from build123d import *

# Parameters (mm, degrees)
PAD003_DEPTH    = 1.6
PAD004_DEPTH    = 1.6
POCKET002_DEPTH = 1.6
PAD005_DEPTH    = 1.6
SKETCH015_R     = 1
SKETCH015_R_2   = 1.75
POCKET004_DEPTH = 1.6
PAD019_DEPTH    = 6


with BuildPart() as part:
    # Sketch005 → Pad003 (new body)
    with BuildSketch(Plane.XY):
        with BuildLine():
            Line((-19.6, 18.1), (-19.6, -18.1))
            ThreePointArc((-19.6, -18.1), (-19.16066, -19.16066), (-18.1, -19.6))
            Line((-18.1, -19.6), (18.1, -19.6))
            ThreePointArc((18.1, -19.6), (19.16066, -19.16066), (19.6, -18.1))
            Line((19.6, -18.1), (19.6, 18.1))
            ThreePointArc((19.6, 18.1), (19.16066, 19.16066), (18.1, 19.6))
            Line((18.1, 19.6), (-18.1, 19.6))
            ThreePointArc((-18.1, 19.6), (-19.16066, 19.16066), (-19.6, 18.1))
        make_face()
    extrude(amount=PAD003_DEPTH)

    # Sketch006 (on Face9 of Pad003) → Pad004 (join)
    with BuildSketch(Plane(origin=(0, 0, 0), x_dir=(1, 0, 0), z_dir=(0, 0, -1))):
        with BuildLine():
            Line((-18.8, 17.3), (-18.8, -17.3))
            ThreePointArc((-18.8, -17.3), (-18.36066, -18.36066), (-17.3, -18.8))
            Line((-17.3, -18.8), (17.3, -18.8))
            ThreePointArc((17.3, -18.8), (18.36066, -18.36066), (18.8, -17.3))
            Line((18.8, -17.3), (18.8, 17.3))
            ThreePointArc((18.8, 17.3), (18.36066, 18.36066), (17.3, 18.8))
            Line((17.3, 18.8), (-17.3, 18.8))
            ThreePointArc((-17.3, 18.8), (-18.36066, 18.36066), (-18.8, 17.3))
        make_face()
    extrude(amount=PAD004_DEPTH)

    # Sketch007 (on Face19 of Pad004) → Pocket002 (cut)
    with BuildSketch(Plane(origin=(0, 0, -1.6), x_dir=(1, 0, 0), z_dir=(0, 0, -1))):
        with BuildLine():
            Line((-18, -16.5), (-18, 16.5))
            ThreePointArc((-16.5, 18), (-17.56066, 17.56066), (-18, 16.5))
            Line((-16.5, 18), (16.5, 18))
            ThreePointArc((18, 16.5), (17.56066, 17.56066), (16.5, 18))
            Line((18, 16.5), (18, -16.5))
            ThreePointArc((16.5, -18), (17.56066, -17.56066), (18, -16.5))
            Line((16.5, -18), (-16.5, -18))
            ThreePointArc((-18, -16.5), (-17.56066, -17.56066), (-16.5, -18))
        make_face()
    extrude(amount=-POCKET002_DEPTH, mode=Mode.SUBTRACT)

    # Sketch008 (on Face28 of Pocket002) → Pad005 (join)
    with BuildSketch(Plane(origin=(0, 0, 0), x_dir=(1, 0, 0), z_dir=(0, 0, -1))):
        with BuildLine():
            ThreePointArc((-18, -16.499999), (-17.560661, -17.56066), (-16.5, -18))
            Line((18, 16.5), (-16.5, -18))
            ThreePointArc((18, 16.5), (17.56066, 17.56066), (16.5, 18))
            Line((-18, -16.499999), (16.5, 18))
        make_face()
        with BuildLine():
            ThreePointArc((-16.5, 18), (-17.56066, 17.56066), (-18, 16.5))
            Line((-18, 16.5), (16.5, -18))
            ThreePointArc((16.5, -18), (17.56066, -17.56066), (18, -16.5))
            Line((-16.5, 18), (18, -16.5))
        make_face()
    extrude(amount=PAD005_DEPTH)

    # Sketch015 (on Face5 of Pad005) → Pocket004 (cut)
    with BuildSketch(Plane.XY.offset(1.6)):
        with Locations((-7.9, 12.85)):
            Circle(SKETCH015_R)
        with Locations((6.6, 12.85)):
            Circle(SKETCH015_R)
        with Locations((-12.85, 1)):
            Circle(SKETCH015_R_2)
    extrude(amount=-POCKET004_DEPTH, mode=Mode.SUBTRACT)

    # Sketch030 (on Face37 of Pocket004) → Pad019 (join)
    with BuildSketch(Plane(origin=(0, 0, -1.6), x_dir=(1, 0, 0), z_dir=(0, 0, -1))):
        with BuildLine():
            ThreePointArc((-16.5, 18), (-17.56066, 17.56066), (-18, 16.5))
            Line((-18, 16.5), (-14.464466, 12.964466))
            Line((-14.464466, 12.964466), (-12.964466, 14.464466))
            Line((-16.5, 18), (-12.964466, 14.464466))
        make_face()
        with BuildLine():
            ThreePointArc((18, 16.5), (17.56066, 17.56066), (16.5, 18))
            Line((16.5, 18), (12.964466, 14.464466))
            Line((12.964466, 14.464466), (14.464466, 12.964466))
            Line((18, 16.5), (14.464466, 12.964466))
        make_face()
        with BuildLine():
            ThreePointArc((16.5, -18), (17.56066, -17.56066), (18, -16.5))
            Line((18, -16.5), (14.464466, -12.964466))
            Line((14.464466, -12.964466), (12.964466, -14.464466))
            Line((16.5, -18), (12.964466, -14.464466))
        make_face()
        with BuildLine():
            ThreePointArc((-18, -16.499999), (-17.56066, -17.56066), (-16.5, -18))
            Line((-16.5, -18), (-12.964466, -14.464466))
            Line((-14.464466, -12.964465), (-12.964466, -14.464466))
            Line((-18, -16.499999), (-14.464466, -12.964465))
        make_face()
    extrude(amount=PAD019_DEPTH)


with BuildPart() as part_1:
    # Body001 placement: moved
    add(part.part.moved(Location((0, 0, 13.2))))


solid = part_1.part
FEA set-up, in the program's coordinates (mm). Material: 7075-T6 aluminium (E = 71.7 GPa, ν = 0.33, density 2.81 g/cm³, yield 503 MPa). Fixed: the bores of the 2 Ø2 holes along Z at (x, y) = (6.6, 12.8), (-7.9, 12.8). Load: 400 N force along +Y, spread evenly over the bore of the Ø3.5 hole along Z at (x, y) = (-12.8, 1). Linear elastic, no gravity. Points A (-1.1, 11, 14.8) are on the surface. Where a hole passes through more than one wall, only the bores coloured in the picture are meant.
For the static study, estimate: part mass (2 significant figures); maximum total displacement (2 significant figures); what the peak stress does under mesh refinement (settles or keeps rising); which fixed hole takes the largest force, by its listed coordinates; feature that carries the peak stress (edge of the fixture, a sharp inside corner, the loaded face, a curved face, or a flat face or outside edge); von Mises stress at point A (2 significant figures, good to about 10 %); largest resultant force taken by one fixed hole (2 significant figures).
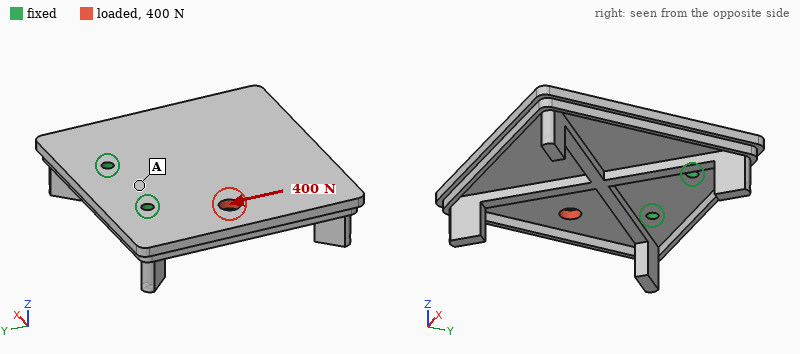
9.0 g
15 µm
keeps rising
(-7.9, 12.8)
edge of the fixture
7.6 MPa
510 N
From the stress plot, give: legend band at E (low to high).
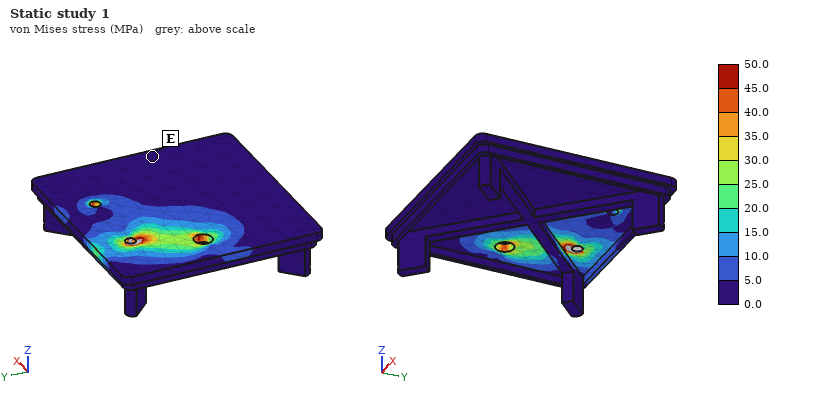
0.0 to 5.0 MPa
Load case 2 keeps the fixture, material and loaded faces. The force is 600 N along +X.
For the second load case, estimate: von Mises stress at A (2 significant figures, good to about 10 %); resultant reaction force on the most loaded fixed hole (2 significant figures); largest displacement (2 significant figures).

28 MPa
560 N
27 µm
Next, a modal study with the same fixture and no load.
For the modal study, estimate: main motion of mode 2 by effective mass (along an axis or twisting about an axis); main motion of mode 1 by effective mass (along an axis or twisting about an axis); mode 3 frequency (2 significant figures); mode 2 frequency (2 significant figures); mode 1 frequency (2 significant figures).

twisting about Y
along Z
6200 Hz
2400 Hz
1200 Hz
